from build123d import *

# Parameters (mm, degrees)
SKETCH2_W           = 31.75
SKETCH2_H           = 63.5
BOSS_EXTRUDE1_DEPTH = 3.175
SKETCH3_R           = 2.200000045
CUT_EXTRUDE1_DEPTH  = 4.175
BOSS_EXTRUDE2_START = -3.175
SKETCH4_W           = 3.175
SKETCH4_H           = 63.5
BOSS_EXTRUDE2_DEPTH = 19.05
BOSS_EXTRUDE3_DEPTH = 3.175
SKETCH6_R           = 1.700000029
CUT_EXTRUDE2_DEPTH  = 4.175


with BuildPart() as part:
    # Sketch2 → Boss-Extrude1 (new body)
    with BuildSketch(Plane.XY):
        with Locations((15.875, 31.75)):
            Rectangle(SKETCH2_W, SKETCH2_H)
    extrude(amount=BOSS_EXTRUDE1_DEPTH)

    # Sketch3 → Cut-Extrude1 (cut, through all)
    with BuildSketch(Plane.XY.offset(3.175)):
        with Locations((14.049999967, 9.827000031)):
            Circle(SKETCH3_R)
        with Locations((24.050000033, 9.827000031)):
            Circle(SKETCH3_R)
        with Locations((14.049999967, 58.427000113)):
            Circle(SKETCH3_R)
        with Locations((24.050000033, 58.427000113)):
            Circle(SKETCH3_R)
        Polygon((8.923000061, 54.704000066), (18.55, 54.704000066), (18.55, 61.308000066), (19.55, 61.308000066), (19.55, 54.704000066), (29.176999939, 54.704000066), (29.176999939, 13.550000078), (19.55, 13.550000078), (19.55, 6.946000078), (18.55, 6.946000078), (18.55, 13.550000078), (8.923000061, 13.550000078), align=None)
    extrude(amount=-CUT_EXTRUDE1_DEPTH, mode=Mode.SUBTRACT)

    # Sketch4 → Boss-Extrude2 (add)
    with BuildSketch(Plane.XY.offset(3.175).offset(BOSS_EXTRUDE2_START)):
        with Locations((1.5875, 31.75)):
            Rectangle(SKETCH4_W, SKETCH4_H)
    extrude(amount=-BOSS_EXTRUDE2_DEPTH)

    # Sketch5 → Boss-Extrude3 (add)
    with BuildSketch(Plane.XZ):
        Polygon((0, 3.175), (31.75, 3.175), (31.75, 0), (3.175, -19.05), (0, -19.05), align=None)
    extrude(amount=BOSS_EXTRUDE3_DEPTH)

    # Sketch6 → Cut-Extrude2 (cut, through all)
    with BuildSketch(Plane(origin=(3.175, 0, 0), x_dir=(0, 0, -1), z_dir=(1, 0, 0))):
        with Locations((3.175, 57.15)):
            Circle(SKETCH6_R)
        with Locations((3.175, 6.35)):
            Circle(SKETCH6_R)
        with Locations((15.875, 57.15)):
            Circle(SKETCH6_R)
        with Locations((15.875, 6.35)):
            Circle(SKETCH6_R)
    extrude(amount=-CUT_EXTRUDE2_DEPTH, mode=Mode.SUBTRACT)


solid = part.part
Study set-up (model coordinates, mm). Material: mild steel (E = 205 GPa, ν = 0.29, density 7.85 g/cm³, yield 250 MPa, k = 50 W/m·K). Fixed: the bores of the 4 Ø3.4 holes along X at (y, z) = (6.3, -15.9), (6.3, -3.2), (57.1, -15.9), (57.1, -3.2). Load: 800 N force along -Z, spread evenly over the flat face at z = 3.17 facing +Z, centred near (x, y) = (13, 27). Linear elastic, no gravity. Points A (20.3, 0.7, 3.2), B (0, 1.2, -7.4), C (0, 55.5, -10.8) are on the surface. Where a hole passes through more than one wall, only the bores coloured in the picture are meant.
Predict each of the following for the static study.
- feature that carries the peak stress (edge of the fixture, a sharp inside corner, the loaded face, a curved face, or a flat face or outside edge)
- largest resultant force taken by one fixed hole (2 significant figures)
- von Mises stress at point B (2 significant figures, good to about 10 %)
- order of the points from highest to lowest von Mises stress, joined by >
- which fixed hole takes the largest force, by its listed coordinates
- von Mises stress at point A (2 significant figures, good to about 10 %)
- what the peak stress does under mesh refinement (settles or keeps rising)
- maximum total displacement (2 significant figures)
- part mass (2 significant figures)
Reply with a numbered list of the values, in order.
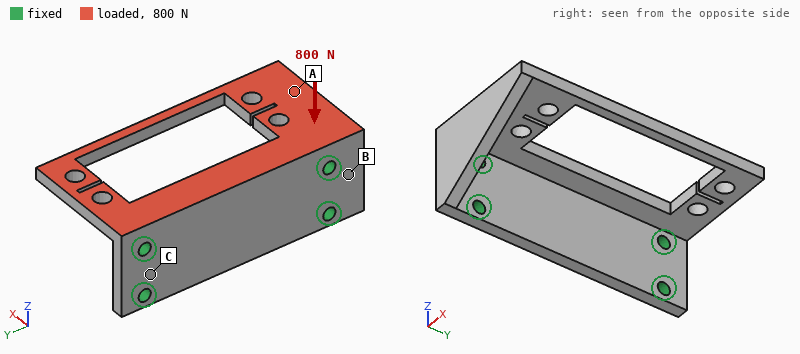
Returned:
1. a sharp inside corner
2. 490 N
3. 32 MPa
4. A > B > C
5. (6.3, -3.2)
6. 53 MPa
7. keeps rising
8. 0.20 mm
9. 68 g
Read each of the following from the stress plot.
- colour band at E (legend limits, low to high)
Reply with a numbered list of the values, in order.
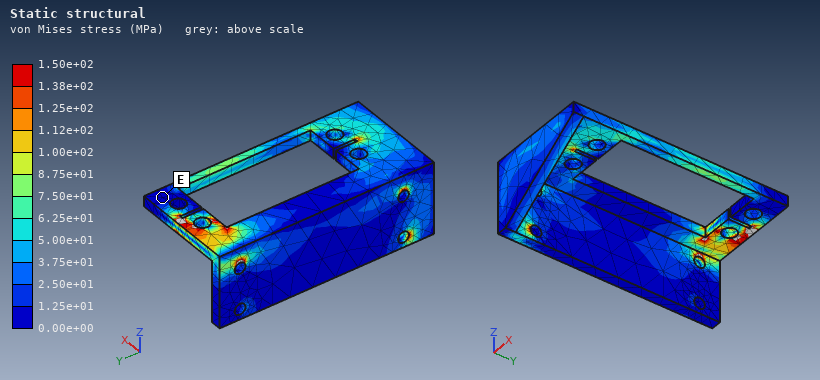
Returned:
1. 0.00e+00 to 1.25e+01 MPa
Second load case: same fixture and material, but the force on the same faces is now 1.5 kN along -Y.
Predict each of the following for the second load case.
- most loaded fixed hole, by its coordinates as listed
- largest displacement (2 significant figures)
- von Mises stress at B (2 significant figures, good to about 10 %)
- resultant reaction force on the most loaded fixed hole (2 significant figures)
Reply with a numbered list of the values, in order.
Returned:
1. (57.1, -3.2)
2. 53 µm
3. 42 MPa
4. 700 N
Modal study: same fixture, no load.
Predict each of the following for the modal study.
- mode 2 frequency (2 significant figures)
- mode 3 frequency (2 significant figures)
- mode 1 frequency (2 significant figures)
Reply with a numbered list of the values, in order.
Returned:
1. 4300 Hz
2. 5100 Hz
3. 2300 Hz
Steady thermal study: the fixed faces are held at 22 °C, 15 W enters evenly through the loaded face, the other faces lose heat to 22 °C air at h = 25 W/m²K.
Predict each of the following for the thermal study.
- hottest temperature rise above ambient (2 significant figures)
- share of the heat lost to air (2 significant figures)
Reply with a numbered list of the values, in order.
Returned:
1. 58 K
2. 15 %
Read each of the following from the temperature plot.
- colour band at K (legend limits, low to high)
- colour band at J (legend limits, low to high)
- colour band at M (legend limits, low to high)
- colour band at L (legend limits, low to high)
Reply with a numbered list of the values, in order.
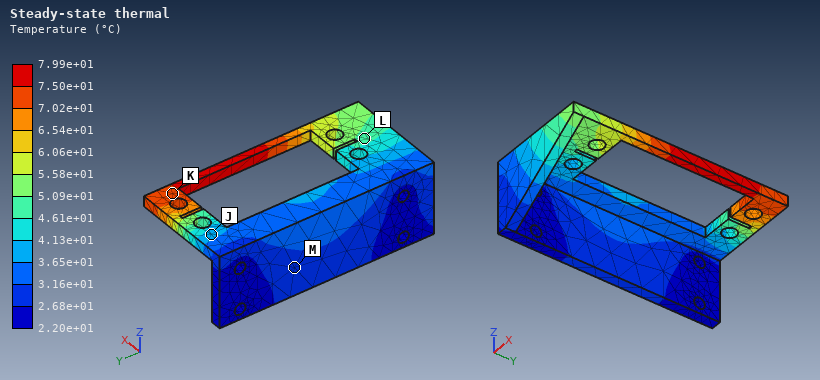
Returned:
1. 7.02e+01 to 7.50e+01 °C
2. 3.65e+01 to 4.13e+01 °C
3. 2.68e+01 to 3.16e+01 °C
4. 4.61e+01 to 5.09e+01 °C
